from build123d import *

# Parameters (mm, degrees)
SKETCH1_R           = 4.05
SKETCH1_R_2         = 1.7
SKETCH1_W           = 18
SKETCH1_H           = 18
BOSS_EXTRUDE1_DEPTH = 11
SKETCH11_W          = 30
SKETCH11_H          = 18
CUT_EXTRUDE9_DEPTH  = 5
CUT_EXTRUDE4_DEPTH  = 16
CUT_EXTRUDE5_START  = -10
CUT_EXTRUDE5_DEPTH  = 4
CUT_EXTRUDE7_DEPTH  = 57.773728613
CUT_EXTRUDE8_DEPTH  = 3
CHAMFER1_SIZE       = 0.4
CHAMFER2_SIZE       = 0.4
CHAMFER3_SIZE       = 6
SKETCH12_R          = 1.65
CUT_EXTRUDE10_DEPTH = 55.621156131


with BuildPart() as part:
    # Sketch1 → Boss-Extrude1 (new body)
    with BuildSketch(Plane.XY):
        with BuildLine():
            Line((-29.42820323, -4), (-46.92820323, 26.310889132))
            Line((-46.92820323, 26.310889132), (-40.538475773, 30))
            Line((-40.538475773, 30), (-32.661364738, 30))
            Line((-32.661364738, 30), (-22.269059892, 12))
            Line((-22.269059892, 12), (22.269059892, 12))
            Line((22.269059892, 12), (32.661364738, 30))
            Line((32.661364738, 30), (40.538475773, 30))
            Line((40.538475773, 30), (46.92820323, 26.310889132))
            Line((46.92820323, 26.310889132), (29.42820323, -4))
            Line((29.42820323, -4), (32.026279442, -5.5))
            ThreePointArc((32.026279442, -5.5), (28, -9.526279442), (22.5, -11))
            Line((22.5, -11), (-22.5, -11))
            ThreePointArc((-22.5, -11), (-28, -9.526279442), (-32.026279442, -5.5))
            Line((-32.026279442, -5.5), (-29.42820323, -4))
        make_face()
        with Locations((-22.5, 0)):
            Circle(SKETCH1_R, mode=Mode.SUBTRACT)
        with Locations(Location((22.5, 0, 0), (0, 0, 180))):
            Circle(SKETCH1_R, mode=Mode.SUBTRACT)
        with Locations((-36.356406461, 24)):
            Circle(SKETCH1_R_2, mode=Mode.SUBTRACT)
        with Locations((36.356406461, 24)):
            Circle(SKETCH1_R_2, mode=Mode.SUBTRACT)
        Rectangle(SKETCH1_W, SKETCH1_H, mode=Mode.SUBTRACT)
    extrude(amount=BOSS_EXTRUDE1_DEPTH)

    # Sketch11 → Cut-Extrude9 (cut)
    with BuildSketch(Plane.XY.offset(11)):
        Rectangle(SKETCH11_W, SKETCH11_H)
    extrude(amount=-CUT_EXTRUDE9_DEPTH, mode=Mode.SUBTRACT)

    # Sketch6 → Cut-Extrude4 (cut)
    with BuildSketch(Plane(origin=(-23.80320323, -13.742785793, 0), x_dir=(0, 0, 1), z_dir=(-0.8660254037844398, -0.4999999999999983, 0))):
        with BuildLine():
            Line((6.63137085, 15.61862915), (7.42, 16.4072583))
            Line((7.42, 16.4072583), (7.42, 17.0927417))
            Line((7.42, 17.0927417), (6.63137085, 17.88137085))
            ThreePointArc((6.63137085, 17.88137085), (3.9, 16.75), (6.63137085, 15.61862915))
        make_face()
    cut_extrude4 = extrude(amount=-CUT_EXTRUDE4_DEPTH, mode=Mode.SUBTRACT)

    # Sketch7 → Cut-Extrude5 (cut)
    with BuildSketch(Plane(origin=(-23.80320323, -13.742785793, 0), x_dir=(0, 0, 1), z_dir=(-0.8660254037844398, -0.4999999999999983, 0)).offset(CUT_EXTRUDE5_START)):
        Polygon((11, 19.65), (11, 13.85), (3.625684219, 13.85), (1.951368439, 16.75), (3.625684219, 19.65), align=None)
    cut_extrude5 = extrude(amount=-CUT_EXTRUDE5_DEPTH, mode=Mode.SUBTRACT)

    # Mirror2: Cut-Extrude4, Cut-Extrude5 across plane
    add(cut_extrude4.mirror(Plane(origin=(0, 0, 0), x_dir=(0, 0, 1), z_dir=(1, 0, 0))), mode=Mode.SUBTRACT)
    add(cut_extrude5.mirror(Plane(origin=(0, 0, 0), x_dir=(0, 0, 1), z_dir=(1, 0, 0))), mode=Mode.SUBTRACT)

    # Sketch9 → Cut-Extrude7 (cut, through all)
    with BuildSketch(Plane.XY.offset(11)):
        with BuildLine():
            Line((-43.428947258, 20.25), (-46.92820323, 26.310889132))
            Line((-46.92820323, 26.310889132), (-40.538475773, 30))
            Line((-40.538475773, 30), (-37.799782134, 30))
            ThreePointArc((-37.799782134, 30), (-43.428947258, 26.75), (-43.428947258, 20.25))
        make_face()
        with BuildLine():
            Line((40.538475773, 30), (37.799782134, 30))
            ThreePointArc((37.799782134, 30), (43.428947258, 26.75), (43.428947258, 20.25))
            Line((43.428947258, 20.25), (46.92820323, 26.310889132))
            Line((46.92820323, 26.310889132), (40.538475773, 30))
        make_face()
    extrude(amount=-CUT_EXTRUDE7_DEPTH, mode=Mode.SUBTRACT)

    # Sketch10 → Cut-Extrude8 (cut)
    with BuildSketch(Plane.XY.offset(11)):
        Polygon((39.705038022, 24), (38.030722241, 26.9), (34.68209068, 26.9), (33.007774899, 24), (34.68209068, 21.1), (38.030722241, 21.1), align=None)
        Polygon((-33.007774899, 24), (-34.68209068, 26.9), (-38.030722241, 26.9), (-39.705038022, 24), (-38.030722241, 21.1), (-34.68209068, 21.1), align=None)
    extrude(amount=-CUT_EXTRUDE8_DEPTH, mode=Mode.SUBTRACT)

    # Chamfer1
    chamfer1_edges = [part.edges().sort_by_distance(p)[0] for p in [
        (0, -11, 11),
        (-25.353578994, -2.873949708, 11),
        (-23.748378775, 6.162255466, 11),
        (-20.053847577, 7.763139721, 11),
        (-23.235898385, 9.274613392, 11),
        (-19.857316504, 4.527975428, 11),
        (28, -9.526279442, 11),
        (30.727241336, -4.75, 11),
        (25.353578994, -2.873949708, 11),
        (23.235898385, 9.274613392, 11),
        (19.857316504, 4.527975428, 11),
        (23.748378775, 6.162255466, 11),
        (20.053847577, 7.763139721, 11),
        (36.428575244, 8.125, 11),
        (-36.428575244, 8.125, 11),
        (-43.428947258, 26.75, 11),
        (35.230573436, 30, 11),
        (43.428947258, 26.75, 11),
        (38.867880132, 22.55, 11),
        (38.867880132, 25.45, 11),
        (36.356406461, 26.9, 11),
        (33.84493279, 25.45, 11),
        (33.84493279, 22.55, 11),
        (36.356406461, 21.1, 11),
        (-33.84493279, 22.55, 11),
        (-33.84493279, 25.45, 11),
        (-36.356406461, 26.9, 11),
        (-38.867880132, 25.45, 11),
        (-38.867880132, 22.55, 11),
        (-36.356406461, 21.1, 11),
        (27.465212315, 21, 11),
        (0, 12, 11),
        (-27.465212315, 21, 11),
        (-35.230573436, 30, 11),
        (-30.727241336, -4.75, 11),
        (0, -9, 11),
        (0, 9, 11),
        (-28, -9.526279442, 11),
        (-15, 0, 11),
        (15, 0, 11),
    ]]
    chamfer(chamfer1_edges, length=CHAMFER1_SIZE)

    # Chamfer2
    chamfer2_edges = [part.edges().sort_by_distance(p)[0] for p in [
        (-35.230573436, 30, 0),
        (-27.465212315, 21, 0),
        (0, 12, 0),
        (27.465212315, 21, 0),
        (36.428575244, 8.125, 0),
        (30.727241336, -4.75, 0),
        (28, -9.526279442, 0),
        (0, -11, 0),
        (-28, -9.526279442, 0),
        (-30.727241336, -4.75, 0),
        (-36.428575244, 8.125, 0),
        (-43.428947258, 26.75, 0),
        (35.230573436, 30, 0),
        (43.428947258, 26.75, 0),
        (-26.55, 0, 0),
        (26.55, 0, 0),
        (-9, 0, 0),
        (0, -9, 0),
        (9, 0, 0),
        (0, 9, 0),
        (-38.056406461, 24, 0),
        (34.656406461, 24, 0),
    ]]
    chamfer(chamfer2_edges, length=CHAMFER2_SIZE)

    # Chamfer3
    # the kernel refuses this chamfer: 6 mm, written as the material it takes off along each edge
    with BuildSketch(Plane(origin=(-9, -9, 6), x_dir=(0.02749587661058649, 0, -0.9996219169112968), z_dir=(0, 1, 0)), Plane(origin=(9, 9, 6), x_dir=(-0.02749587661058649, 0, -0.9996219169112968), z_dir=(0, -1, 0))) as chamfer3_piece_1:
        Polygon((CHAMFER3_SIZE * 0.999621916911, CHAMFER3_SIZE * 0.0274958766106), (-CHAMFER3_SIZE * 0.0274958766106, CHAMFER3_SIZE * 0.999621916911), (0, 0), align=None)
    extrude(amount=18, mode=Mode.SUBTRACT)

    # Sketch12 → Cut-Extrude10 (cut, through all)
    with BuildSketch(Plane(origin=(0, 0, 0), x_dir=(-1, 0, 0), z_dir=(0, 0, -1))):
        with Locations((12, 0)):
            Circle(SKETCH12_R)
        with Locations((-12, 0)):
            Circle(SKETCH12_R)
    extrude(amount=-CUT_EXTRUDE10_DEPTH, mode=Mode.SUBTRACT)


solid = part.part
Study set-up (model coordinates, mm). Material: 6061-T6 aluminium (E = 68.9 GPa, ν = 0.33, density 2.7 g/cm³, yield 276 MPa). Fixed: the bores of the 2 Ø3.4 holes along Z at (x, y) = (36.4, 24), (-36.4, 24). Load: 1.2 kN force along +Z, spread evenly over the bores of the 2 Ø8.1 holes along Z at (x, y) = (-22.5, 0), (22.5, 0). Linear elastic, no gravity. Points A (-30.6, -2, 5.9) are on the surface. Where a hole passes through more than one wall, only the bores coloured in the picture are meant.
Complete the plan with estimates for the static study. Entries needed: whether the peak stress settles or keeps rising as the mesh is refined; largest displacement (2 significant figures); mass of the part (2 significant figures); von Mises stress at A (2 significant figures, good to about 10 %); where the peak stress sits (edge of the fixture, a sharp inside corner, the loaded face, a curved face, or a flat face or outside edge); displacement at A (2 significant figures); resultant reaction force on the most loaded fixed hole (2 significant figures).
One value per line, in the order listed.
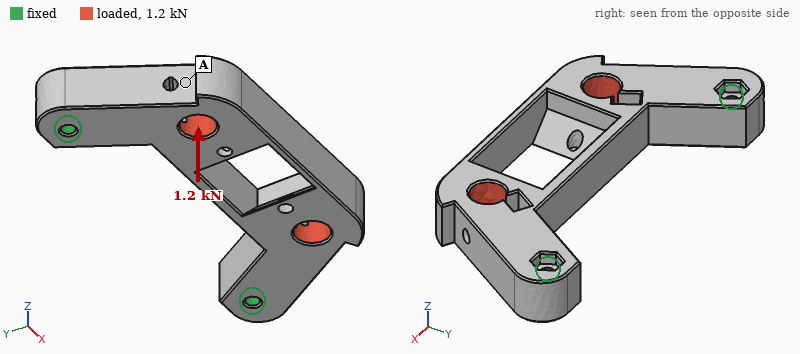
keeps rising
0.12 mm
40 g
22 MPa
edge of the fixture
0.065 mm
600 N
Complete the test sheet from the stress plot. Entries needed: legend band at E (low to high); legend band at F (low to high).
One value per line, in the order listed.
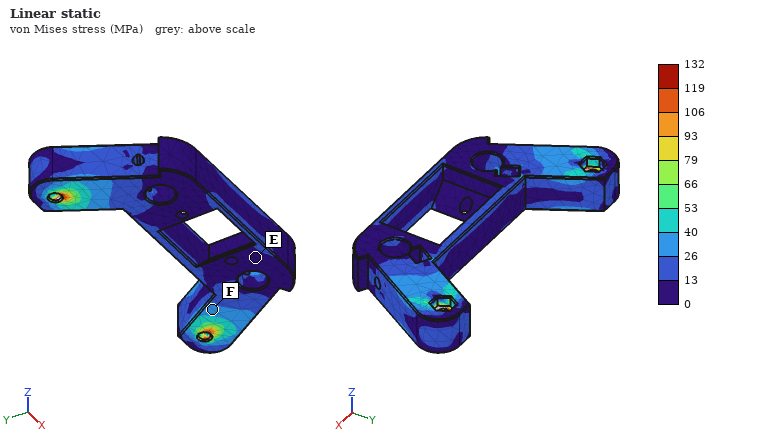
0 to 13 MPa
26 to 40 MPa
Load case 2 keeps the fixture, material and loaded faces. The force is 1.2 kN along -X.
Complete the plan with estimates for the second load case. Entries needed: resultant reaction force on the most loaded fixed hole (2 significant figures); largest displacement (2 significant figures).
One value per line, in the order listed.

620 N
67 µm
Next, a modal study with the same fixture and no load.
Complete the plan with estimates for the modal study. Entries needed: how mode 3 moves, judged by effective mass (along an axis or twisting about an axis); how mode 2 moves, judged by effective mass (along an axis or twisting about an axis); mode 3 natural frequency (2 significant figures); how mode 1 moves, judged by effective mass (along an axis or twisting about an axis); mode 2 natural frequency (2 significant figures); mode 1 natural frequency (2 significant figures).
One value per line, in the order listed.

twisting about Y
along X
6700 Hz
along Z
4700 Hz
4000 Hz
